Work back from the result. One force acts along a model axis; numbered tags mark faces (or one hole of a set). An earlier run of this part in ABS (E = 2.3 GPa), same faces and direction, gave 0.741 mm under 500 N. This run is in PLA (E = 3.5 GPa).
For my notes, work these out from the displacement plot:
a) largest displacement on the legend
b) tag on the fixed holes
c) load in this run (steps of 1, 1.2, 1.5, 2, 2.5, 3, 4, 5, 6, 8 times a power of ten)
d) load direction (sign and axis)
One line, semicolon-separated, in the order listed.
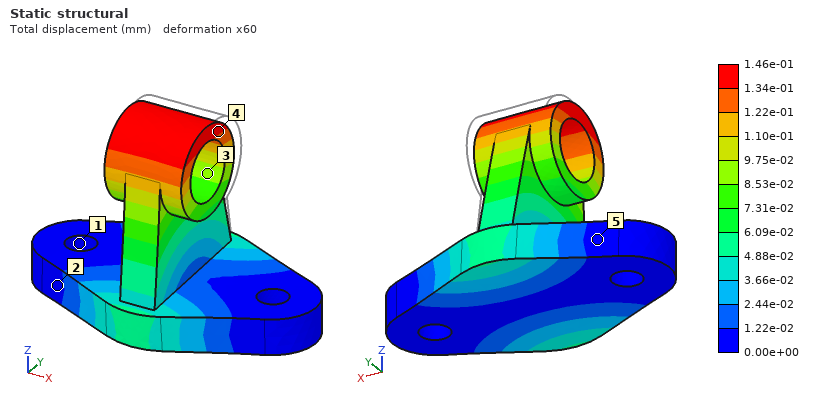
1.46e-01 mm; 1; 150 N; -Y
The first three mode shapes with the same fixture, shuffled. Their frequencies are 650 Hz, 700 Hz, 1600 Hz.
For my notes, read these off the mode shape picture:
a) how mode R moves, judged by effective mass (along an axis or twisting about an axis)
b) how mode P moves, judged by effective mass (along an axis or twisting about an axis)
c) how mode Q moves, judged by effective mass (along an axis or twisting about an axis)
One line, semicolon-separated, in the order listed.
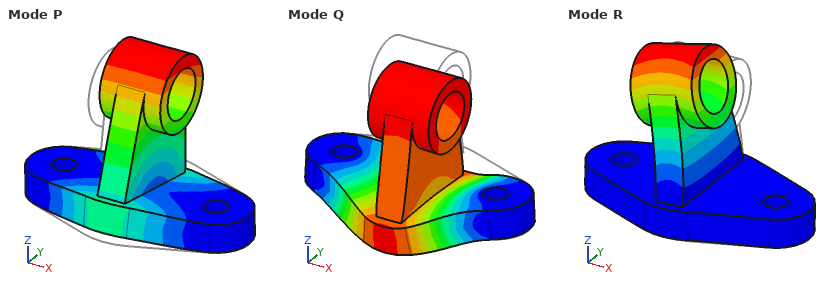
along X; along Y; along Z
